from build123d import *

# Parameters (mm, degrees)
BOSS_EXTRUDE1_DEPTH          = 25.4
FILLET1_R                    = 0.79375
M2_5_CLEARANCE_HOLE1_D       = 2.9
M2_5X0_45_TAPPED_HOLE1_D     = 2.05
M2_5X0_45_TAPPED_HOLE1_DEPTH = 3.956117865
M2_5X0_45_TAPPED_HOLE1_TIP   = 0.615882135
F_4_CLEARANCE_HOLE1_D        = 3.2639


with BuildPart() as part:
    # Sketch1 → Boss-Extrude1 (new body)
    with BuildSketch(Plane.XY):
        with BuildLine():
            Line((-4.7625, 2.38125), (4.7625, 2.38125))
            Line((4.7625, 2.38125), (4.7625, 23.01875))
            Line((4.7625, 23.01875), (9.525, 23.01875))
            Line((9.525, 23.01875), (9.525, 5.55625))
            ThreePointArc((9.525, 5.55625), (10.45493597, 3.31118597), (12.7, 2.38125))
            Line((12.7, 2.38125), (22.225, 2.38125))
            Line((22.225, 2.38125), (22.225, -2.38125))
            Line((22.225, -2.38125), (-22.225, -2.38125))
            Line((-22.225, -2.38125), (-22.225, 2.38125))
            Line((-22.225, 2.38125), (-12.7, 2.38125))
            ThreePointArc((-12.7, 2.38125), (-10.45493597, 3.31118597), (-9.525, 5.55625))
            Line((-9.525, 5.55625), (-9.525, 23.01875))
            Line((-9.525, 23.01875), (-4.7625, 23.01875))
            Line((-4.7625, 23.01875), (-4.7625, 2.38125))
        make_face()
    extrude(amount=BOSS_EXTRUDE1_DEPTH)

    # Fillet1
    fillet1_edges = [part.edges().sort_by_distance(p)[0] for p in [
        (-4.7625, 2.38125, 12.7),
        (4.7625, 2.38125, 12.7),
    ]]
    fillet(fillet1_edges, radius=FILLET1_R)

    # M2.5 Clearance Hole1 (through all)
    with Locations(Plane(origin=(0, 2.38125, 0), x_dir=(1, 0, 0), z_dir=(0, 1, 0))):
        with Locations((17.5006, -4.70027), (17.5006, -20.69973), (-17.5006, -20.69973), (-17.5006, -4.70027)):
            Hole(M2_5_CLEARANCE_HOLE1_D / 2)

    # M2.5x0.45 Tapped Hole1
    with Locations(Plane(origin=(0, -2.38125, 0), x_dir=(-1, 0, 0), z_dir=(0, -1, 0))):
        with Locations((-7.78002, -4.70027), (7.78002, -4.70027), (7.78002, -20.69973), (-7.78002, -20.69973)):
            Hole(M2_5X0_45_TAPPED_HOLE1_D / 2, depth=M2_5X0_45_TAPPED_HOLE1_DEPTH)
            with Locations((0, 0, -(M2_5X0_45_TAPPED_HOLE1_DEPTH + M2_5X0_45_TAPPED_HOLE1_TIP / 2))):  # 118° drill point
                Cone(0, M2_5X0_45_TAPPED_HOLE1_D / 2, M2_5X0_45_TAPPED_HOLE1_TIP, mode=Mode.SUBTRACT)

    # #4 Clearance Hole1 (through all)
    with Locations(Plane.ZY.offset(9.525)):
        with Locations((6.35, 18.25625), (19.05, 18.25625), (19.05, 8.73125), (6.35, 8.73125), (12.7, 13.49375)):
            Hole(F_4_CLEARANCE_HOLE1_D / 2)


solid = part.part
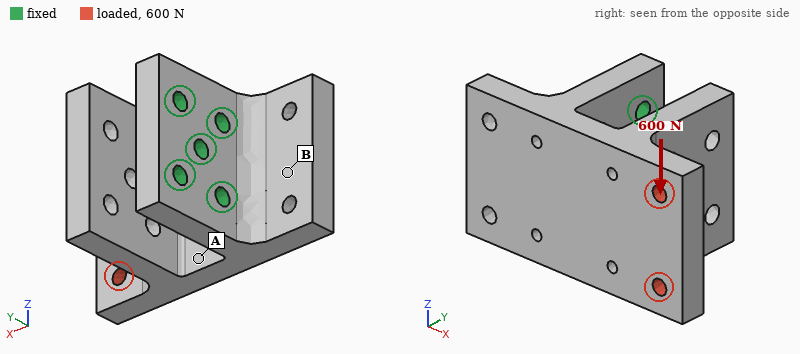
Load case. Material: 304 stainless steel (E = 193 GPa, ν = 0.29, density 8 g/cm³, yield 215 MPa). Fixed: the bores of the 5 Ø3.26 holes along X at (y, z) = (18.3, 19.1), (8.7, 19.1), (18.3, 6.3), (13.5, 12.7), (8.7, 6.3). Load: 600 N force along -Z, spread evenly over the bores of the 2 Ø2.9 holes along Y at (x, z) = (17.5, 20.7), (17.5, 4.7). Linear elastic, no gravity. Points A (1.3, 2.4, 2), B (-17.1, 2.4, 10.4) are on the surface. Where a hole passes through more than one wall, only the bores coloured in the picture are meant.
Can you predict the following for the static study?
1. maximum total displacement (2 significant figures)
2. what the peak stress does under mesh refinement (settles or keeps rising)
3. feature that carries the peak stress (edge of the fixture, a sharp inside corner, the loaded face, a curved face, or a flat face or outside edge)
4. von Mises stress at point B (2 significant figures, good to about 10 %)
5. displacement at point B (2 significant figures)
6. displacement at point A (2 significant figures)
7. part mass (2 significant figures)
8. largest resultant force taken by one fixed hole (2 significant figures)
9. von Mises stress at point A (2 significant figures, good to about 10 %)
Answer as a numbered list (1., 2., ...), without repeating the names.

1. 23 µm
2. keeps rising
3. edge of the fixture
4. 11 MPa
5. 5.0 µm
6. 9.1 µm
7. 79 g
8. 990 N
9. 31 MPa
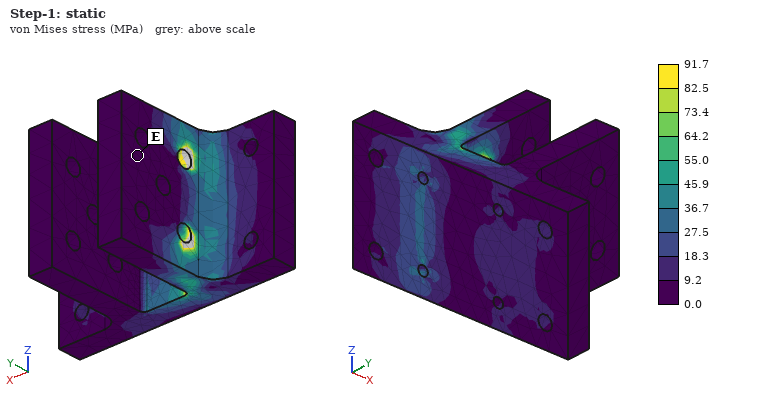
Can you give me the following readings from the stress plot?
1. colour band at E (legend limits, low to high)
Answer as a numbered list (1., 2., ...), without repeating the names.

1. 0.0 to 9.2 MPa
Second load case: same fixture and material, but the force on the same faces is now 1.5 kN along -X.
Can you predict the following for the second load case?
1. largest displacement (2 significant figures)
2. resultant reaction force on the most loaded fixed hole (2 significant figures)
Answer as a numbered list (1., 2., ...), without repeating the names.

1. 39 µm
2. 900 N
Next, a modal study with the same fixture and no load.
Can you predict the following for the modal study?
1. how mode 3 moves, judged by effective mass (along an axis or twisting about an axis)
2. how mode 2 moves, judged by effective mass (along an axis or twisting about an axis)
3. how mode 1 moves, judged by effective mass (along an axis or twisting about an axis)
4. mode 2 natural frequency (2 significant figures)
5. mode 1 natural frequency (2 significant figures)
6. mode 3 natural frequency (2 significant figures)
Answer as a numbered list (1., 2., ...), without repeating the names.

1. along X
2. along Z
3. along Y
4. 4800 Hz
5. 2400 Hz
6. 6500 Hz
